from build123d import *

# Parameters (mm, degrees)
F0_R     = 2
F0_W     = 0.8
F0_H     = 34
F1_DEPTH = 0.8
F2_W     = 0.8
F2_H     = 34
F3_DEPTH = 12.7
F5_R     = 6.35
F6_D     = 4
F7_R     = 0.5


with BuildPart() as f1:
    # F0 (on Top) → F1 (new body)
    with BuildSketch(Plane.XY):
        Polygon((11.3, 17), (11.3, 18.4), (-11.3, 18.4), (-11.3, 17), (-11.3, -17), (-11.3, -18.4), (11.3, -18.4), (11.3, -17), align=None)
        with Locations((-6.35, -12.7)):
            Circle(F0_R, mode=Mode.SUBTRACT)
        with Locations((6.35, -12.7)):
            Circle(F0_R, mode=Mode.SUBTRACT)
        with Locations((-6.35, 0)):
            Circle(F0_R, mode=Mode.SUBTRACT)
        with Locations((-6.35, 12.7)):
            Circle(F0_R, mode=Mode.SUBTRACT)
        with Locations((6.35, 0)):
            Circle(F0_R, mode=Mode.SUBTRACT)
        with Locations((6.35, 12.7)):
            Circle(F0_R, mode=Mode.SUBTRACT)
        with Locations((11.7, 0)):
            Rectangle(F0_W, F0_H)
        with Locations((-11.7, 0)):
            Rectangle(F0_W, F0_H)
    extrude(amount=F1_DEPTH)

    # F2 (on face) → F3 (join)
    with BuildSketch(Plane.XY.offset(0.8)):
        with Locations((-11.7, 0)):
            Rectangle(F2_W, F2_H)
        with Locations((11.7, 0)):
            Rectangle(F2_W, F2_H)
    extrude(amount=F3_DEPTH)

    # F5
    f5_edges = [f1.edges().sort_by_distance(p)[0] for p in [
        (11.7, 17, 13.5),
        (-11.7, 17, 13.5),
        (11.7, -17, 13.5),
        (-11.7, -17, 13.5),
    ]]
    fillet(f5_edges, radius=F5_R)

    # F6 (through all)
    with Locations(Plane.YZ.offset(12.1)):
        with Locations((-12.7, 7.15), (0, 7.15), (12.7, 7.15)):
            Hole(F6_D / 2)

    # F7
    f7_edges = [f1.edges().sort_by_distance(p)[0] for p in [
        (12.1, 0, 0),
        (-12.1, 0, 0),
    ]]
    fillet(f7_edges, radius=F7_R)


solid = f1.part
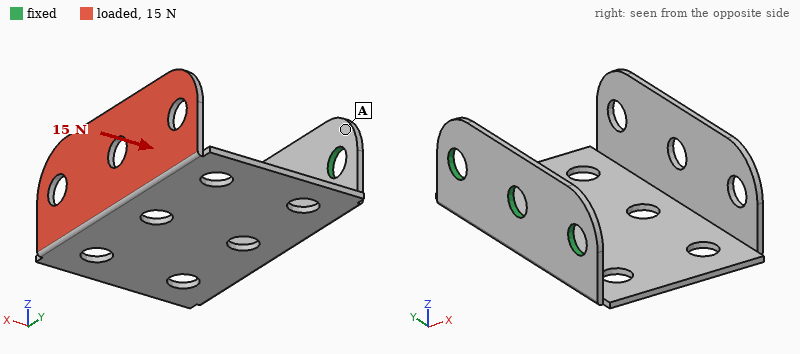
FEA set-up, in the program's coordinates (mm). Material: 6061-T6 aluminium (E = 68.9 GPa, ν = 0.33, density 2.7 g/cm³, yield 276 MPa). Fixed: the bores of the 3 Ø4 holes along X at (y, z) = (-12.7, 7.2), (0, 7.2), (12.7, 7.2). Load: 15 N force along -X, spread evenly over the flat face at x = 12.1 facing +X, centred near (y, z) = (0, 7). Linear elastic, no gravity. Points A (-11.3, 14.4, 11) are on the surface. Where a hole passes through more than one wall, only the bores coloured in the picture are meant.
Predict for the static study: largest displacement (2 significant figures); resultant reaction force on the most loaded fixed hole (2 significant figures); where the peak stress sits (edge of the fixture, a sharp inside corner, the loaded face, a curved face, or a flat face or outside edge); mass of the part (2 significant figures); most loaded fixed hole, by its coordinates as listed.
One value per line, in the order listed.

0.50 mm
5.6 N
a curved face
3.4 g
(0, 7.2)
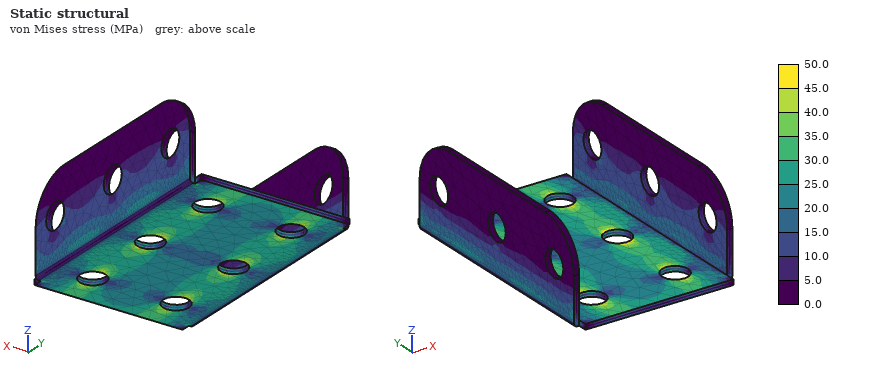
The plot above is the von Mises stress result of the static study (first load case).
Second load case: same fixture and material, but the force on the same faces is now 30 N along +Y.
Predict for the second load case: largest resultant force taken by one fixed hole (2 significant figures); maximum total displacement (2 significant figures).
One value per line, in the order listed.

29 N
0.50 mm
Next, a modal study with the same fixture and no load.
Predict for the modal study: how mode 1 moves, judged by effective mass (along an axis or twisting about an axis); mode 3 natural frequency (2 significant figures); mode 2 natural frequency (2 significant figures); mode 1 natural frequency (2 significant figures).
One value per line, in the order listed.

along Z
2000 Hz
1100 Hz
510 Hz
